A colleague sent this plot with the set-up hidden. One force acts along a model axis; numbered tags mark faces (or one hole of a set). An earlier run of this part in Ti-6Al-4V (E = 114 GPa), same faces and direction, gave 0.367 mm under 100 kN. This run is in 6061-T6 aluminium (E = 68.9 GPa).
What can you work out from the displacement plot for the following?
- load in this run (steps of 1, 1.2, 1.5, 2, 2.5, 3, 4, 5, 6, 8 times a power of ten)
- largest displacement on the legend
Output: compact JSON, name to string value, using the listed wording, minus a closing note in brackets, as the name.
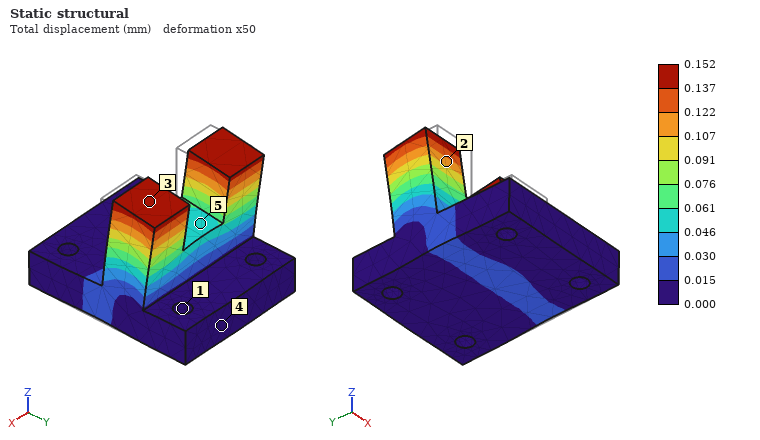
{"load in this run": "25 kN", "largest displacement on the legend": "0.152 mm"}
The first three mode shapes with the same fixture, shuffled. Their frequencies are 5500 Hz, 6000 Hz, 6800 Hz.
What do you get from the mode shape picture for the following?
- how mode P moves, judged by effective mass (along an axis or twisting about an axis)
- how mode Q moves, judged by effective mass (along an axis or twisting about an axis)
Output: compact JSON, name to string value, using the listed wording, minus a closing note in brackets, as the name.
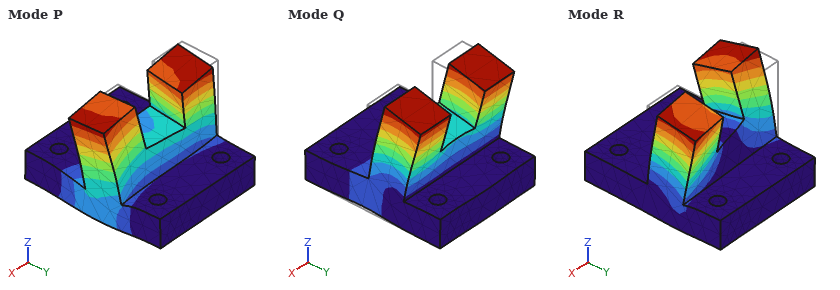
{"how mode P moves, judged by effective mass": "along X", "how mode Q moves, judged by effective mass": "along Y"}
